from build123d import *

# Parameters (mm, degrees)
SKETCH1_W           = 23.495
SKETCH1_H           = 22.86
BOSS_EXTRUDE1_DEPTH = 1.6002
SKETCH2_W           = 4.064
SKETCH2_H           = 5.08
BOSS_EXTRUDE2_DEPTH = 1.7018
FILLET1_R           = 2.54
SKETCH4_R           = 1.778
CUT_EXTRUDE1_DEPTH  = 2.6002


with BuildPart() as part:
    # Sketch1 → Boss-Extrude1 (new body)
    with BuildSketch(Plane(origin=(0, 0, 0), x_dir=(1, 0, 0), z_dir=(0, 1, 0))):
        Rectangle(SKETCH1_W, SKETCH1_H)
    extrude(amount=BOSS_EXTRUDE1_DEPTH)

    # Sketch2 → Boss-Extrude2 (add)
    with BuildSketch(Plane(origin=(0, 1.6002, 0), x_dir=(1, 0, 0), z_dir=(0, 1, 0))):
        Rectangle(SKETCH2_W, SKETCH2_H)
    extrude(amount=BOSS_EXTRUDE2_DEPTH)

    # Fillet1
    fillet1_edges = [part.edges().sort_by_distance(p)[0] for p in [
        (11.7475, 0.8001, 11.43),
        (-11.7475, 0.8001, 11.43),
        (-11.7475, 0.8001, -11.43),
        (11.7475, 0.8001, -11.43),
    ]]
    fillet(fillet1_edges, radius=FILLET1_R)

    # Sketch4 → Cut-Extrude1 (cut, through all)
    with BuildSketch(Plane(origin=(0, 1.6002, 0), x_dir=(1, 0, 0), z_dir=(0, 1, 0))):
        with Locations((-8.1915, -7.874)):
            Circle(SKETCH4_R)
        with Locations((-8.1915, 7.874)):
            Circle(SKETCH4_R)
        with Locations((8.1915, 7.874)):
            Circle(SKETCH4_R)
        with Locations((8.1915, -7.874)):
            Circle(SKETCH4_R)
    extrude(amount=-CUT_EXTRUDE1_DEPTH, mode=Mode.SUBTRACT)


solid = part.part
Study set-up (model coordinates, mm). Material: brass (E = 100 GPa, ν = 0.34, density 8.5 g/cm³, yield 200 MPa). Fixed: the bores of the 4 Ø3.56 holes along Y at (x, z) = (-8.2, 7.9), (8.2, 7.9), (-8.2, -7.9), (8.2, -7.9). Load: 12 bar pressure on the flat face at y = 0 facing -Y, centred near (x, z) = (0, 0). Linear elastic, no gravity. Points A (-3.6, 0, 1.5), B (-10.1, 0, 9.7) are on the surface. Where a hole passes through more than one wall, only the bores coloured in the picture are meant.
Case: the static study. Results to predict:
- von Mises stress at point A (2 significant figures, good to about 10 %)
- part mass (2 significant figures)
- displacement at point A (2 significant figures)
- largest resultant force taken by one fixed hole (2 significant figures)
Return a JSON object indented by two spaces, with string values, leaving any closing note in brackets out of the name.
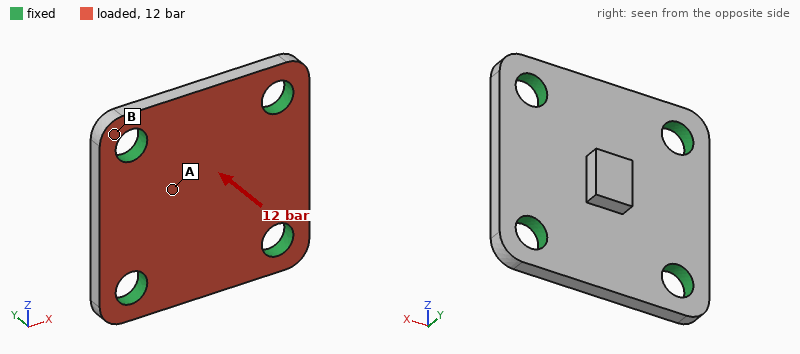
{
  "von Mises stress at point A": "19 MPa",
  "part mass": "7.0 g",
  "displacement at point A": "6.2 µm",
  "largest resultant force taken by one fixed hole": "150 N"
}
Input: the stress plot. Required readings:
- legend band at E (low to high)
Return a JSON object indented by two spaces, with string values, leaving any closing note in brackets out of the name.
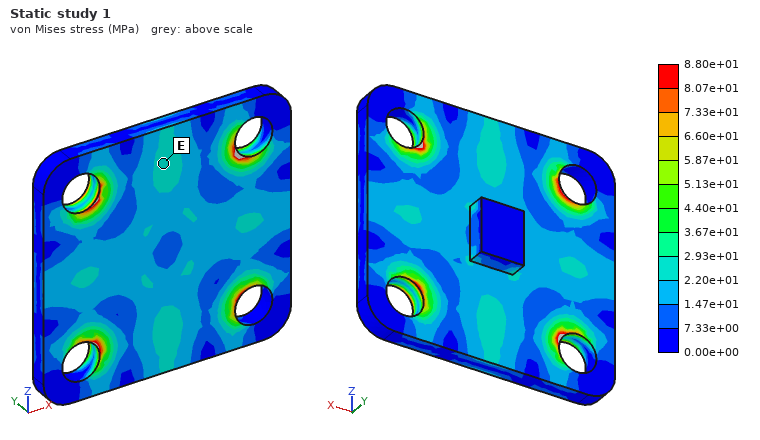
{
  "legend band at E": "2.20e+01 to 2.93e+01 MPa"
}
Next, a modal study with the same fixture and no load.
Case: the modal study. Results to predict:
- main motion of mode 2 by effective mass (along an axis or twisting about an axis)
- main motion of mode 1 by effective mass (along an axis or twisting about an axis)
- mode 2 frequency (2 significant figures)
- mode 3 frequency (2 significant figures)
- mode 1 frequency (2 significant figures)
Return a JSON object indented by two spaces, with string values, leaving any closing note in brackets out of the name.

{
  "main motion of mode 2 by effective mass": "twisting about X",
  "main motion of mode 1 by effective mass": "along Y",
  "mode 2 frequency": "28 kHz",
  "mode 3 frequency": "30 kHz",
  "mode 1 frequency": "19 kHz"
}
